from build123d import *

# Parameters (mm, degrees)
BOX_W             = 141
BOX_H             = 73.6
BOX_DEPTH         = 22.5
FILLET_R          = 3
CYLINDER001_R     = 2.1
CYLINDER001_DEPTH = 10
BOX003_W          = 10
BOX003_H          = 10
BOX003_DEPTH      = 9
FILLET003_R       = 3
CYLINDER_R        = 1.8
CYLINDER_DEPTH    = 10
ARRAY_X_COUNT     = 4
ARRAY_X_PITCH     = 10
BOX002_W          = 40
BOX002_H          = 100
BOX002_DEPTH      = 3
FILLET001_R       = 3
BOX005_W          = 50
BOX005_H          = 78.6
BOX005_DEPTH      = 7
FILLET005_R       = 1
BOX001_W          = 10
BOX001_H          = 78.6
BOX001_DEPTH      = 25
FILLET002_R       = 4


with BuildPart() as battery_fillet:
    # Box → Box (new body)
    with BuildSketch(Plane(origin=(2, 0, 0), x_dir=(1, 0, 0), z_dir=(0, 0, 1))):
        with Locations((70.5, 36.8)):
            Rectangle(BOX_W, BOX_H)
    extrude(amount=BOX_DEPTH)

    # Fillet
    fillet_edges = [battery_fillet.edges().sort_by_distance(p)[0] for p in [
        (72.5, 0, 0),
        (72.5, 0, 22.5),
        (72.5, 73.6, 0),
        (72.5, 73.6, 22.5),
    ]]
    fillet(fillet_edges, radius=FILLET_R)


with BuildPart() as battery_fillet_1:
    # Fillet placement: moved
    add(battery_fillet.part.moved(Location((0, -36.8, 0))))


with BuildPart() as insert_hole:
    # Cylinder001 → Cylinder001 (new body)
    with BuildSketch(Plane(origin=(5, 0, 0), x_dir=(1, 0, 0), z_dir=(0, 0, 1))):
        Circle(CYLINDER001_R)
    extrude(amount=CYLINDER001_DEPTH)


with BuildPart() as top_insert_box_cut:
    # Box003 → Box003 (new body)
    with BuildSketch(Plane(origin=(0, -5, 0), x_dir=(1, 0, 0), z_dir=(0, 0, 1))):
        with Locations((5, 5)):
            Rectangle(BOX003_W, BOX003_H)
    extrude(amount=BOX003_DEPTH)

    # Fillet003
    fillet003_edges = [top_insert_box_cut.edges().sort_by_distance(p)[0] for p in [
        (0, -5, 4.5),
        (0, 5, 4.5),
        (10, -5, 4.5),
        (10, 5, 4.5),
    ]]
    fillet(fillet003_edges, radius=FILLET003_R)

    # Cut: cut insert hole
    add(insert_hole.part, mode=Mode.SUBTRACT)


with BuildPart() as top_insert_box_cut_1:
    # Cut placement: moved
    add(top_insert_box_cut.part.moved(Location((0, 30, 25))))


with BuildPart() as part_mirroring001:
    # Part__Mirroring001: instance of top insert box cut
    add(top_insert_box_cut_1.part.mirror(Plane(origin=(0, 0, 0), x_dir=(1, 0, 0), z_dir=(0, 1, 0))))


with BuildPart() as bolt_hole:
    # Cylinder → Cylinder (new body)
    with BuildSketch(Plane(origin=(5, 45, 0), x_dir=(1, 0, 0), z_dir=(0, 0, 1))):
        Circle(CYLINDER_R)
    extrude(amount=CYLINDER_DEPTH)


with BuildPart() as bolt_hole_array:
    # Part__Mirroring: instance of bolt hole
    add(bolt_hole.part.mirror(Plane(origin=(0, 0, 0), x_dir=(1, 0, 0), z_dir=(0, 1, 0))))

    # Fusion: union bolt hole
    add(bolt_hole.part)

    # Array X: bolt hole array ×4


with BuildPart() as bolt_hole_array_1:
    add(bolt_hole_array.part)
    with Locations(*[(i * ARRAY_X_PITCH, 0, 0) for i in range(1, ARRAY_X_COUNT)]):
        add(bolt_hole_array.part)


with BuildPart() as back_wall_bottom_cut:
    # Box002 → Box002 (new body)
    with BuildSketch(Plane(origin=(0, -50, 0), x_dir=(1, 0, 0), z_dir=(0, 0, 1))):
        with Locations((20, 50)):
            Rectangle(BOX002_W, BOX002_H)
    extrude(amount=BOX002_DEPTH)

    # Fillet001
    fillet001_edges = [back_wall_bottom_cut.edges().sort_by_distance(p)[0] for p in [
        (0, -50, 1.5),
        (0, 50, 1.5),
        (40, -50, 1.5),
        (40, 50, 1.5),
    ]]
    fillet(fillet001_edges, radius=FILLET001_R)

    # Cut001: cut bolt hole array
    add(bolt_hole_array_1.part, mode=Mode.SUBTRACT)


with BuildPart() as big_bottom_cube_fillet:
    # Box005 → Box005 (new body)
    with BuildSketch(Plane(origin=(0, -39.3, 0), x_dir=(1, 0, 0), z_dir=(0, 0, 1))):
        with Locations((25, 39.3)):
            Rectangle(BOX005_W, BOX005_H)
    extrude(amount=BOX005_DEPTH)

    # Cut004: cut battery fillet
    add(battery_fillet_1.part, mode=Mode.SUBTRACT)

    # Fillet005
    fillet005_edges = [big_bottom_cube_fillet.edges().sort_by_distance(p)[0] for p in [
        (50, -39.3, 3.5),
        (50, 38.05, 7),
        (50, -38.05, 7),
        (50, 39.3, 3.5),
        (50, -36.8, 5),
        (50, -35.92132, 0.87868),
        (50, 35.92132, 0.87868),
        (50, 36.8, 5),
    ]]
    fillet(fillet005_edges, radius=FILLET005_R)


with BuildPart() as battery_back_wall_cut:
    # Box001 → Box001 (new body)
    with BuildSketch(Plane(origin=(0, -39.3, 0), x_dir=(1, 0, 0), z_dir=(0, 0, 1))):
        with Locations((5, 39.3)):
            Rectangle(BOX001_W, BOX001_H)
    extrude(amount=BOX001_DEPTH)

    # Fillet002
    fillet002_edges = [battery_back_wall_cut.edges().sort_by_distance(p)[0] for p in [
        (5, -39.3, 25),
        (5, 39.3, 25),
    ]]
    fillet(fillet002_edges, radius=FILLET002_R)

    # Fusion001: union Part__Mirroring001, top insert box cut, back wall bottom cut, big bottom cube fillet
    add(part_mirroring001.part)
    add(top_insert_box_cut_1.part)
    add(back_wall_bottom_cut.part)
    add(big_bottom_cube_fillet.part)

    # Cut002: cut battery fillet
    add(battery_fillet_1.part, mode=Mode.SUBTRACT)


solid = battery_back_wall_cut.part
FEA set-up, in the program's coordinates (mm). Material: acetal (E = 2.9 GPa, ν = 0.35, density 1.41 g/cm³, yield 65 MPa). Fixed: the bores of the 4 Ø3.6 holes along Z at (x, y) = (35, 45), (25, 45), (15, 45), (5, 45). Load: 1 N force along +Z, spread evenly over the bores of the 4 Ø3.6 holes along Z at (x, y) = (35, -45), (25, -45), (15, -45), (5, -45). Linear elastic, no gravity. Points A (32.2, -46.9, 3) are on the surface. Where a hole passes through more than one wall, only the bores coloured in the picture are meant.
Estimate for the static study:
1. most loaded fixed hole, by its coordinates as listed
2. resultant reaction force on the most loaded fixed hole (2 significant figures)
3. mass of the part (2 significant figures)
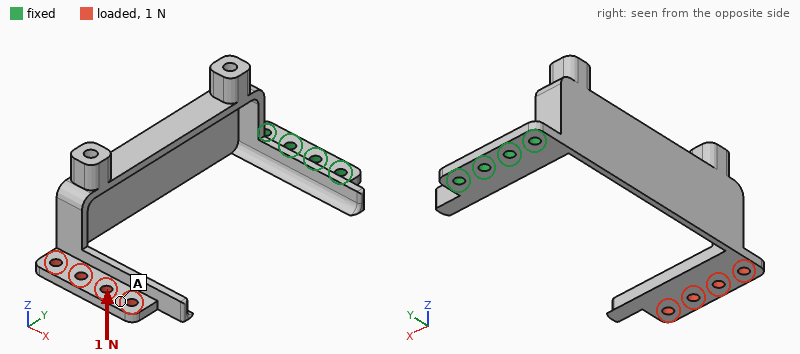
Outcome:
(15, 45)
2.4 N
16 g
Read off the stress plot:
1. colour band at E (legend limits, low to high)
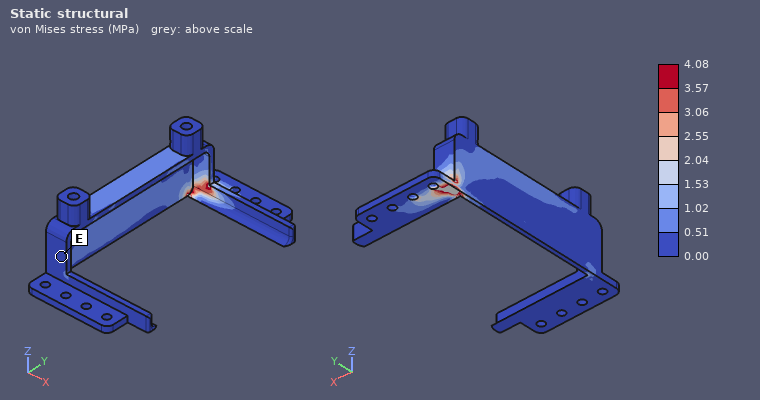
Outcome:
0.00 to 0.51 MPa
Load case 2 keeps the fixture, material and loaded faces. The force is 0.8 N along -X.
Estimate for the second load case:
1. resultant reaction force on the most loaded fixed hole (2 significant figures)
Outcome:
5.9 N
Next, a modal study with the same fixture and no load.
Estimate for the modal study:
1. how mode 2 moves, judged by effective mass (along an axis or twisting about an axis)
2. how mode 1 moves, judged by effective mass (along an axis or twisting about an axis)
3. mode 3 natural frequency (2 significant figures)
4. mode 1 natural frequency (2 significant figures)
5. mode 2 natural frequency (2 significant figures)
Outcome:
along Z
along X
170 Hz
54 Hz
72 Hz
